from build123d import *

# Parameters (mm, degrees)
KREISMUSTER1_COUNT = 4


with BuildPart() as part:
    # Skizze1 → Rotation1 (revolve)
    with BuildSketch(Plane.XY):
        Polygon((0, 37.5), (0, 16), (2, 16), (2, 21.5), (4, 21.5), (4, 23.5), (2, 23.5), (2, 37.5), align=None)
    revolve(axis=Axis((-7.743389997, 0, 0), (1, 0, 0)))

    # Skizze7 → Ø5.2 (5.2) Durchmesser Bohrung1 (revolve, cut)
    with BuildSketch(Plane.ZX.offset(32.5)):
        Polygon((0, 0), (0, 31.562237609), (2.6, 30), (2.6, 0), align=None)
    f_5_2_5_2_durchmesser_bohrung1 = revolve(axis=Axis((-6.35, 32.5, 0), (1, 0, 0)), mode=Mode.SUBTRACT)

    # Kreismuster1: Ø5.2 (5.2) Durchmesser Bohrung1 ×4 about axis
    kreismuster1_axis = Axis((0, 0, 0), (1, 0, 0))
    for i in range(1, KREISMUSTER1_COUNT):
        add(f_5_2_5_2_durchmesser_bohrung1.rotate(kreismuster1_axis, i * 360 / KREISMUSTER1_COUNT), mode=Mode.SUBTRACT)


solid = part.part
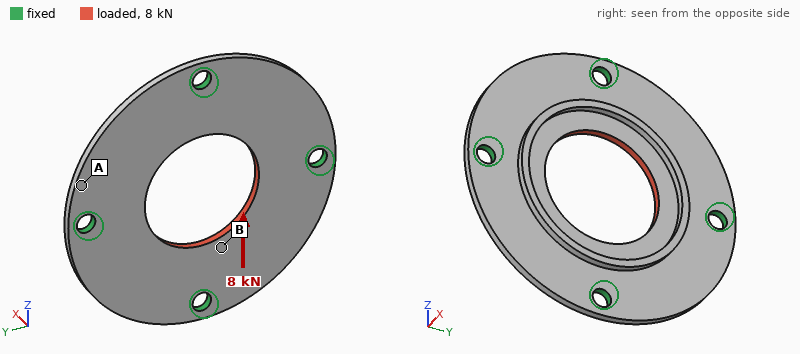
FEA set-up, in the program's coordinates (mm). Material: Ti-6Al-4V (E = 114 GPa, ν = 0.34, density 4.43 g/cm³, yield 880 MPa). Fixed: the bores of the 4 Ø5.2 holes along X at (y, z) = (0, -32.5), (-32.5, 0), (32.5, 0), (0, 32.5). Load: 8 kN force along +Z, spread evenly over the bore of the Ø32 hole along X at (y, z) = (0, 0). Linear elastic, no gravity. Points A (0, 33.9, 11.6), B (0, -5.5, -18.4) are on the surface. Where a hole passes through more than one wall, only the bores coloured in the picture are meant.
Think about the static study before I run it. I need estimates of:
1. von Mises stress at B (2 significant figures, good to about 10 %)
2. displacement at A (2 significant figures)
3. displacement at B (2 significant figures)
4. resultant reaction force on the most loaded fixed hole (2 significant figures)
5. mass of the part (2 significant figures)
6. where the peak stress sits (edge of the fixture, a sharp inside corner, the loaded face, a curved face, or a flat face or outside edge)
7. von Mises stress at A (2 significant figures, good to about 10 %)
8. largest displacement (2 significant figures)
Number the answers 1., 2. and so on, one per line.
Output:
1. 64 MPa
2. 4.5 µm
3. 9.6 µm
4. 2.2 kN
5. 34 g
6. edge of the fixture
7. 31 MPa
8. 15 µm
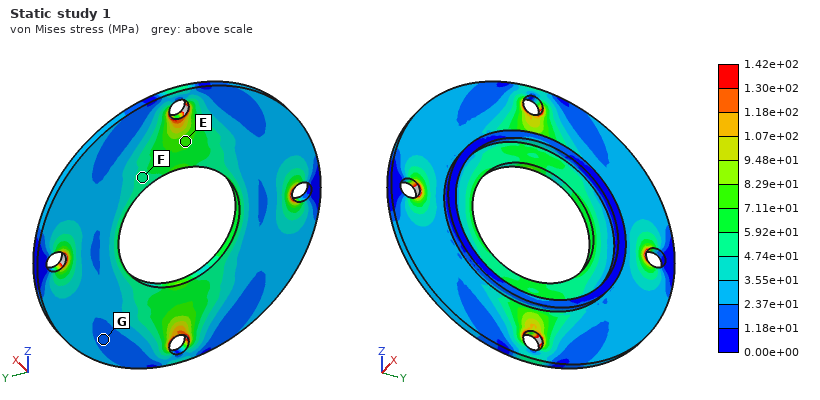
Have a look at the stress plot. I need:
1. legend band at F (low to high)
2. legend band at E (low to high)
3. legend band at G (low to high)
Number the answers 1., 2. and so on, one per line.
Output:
1. 4.74e+01 to 5.92e+01 MPa
2. 7.11e+01 to 8.29e+01 MPa
3. 1.18e+01 to 2.37e+01 MPa
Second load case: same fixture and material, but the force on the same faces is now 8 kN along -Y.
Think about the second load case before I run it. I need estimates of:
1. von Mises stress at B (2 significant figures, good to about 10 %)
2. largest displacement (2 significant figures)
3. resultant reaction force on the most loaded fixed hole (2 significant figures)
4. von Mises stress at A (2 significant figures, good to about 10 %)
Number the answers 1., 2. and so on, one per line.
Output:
1. 32 MPa
2. 15 µm
3. 2.2 kN
4. 17 MPa
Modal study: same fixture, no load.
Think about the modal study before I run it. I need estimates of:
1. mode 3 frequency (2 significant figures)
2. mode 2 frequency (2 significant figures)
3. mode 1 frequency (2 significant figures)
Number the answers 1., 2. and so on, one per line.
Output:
1. 5100 Hz
2. 5100 Hz
3. 4700 Hz
